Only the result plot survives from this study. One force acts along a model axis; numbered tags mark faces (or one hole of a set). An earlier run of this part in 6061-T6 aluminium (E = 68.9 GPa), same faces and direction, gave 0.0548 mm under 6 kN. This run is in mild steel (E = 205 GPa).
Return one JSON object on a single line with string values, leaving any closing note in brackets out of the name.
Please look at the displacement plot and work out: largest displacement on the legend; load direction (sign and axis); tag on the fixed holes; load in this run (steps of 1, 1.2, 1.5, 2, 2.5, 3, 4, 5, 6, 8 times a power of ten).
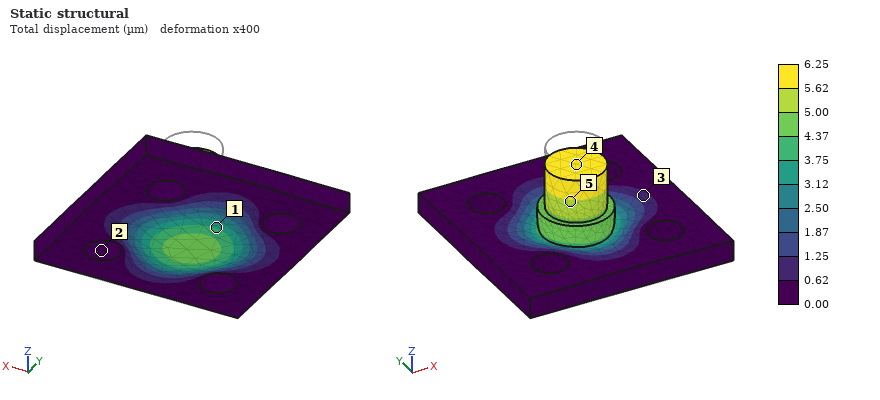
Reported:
{"largest displacement on the legend": "6.25 µm", "load direction": "-Z", "tag on the fixed holes": "2", "load in this run": "2 kN"}
